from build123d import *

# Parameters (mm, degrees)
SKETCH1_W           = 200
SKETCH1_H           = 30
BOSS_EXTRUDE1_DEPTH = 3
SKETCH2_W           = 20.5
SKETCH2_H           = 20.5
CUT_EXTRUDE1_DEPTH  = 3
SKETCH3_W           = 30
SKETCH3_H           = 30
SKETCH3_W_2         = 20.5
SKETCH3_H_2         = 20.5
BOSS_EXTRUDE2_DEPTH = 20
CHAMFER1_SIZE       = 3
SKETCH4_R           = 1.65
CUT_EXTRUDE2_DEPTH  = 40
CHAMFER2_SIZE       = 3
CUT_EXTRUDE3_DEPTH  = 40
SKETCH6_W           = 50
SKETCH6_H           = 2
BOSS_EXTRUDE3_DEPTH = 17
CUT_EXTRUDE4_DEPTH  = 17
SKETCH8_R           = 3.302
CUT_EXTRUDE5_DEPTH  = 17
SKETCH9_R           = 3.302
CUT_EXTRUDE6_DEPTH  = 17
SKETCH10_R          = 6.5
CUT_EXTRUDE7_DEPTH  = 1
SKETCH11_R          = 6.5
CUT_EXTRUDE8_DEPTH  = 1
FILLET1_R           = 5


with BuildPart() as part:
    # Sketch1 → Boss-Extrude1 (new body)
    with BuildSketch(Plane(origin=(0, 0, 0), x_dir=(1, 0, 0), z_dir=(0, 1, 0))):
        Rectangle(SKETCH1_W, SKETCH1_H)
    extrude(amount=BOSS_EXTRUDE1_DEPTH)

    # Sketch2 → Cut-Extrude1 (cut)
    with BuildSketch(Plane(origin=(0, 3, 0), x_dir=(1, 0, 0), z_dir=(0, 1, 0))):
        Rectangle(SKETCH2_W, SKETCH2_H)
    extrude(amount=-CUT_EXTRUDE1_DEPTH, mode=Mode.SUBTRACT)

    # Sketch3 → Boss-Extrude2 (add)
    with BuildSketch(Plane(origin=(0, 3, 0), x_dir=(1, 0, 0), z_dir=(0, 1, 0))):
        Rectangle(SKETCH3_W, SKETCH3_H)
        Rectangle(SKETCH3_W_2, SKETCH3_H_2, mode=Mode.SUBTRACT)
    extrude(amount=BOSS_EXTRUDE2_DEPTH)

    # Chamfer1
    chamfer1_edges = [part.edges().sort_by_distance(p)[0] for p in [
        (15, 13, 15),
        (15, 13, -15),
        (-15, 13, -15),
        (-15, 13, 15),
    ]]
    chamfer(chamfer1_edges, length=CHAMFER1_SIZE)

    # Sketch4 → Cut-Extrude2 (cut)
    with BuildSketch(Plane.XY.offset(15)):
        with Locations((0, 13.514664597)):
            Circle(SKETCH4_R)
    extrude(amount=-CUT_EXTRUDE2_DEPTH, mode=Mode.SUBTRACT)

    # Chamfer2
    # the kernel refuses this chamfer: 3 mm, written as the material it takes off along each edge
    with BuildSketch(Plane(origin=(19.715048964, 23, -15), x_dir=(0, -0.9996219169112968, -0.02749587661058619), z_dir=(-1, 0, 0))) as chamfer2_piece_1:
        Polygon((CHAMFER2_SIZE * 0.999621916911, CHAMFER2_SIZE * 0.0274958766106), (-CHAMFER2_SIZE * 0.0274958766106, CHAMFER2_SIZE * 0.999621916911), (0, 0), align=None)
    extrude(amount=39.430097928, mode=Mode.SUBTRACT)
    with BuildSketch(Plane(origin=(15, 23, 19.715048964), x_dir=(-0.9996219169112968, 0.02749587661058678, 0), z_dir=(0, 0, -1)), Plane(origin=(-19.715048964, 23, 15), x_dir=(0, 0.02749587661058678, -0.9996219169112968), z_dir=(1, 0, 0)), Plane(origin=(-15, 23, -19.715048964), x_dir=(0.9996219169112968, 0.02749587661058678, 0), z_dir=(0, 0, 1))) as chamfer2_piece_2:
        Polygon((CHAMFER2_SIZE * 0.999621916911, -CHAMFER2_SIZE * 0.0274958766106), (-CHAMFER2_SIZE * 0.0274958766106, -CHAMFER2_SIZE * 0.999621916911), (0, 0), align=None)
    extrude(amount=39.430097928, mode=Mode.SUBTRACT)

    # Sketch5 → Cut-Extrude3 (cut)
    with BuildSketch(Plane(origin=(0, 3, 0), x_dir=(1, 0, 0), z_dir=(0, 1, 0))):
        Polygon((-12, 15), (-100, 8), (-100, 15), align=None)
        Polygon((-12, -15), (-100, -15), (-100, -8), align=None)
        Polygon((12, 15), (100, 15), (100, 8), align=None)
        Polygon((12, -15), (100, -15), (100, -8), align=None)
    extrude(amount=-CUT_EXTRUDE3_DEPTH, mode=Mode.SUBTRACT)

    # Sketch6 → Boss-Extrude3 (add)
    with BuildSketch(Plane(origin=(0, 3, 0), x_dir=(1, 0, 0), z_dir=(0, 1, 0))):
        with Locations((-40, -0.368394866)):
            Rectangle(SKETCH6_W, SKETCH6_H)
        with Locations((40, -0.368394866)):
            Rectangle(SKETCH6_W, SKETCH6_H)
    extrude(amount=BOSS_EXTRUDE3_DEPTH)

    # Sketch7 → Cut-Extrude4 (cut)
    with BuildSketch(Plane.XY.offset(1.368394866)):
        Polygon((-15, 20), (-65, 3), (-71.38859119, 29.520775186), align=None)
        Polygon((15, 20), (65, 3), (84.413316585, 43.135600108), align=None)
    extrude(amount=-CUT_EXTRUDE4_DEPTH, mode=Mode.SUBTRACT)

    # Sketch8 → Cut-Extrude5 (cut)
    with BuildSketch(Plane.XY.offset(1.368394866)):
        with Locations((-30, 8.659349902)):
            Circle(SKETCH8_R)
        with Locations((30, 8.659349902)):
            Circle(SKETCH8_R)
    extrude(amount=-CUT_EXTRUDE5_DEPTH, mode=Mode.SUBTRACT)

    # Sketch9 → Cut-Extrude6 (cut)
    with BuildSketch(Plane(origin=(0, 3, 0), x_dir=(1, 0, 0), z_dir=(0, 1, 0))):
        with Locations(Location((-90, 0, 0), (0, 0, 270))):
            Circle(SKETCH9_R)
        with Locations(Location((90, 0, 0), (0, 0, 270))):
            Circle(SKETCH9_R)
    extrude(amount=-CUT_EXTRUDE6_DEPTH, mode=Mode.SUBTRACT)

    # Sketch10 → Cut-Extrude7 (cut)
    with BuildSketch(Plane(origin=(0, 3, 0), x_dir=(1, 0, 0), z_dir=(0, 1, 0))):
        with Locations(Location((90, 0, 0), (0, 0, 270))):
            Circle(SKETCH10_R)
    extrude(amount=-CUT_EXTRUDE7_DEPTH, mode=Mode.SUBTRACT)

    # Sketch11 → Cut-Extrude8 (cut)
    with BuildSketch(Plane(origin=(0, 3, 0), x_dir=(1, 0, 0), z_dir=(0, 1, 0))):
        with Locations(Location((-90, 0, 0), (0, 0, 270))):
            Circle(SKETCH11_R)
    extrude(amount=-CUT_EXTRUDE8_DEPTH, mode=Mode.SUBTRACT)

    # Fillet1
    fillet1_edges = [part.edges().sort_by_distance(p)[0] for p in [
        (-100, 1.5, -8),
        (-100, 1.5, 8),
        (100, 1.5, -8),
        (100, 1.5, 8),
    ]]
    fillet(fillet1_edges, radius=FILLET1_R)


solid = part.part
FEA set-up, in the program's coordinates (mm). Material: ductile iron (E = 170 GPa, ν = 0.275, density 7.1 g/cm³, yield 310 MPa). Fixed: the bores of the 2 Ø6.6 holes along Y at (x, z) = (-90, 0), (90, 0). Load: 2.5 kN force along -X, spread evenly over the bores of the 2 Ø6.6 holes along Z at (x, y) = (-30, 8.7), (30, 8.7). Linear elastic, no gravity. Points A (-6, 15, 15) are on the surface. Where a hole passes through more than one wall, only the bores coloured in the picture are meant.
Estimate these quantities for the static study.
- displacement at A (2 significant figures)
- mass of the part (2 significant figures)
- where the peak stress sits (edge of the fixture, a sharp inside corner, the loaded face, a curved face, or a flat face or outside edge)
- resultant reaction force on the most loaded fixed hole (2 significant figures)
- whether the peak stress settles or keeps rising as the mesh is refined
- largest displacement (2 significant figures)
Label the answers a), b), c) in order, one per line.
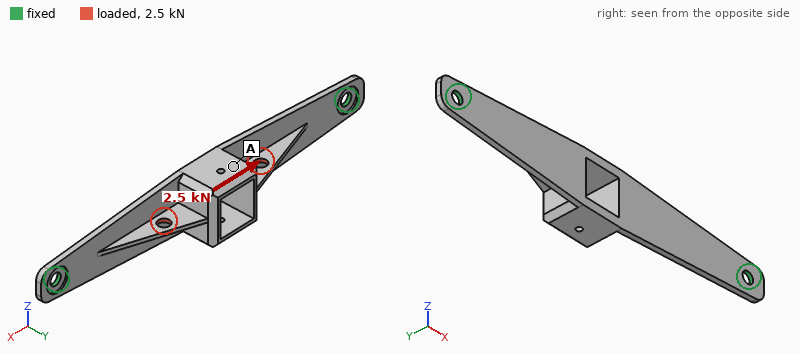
a) 19 µm
b) 160 g
c) edge of the fixture
d) 1.3 kN
e) keeps rising
f) 45 µm
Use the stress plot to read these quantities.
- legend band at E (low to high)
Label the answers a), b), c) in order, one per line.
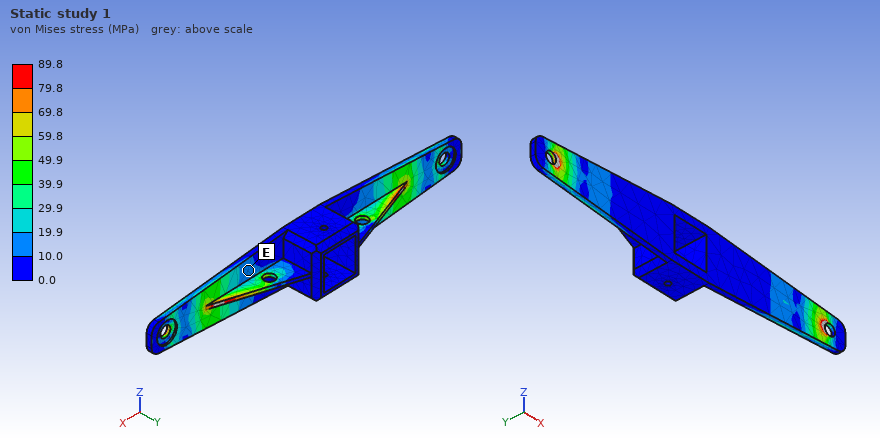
a) 10.0 to 19.9 MPa
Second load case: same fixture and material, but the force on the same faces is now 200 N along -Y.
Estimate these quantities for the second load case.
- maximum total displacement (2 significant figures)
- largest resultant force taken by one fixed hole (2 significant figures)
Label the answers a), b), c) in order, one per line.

a) 97 µm
b) 290 N
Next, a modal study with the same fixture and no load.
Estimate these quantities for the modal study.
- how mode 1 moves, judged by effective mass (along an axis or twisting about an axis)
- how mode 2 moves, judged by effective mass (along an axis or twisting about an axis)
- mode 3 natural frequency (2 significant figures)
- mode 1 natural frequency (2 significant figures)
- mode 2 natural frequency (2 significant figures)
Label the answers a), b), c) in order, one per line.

a) along Y
b) along Z
c) 1800 Hz
d) 630 Hz
e) 680 Hz
